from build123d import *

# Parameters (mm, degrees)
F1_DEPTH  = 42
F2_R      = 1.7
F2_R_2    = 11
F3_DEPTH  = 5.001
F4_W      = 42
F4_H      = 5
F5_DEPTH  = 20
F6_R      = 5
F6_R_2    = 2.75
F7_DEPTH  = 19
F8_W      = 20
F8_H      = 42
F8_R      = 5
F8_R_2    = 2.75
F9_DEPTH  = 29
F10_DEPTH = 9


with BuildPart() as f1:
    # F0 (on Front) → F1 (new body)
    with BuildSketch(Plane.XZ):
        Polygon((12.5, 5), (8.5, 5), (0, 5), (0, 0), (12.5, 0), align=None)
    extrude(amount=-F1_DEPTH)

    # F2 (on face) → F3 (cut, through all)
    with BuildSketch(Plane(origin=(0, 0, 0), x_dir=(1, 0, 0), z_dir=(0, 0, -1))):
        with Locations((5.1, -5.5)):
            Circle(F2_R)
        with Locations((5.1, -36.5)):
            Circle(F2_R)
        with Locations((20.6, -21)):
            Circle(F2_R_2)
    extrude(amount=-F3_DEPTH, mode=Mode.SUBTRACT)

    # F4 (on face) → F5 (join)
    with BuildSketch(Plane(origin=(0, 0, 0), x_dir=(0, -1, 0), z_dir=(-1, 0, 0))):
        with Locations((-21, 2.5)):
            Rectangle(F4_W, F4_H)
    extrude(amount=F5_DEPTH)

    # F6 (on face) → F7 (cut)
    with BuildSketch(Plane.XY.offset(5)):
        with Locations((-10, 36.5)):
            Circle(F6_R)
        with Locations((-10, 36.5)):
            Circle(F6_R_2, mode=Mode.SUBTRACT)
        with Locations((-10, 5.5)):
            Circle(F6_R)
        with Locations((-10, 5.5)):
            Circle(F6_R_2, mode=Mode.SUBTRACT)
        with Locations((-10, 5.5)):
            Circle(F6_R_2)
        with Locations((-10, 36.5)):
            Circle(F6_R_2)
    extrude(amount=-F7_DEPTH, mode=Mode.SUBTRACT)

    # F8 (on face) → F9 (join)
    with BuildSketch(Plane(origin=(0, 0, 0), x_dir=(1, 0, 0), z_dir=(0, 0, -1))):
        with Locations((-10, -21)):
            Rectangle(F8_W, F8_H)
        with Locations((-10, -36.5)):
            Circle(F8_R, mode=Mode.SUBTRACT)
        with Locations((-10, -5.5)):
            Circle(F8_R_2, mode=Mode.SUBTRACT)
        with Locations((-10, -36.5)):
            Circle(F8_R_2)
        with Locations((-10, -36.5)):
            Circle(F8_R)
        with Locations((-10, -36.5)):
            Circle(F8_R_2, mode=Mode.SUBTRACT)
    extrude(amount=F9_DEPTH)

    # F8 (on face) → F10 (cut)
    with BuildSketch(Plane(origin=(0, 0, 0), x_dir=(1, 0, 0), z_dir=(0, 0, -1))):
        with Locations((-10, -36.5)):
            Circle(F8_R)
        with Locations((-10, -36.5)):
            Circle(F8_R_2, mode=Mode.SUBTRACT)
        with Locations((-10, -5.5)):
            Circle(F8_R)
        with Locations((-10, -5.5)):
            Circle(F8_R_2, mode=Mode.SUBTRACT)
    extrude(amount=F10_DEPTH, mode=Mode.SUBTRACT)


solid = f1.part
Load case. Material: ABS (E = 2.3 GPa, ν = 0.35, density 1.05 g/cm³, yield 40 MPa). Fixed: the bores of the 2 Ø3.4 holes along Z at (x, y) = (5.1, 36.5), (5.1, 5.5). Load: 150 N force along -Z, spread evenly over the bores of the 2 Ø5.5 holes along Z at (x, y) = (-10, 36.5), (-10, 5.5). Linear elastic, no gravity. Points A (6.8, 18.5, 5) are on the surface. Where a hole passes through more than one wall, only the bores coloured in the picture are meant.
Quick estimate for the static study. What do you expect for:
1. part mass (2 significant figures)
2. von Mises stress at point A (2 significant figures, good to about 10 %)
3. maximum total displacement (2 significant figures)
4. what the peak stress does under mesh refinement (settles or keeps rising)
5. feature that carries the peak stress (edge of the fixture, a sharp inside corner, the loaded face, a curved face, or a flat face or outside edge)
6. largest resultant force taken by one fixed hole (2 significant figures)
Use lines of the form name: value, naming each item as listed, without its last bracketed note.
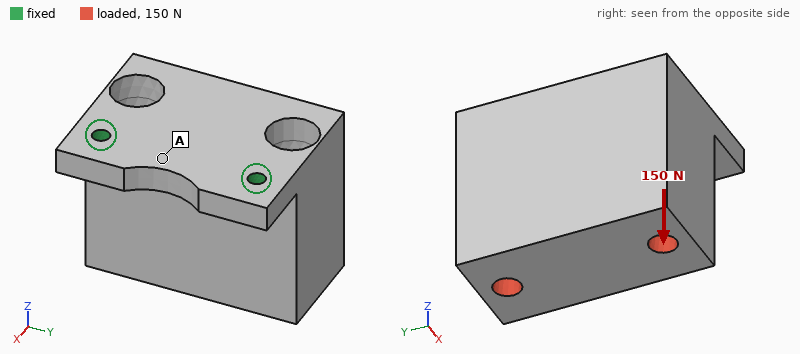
part mass: 29 g
von Mises stress at point A: 2.9 MPa
maximum total displacement: 0.67 mm
what the peak stress does under mesh refinement: keeps rising
feature that carries the peak stress: edge of the fixture
largest resultant force taken by one fixed hole: 75 N
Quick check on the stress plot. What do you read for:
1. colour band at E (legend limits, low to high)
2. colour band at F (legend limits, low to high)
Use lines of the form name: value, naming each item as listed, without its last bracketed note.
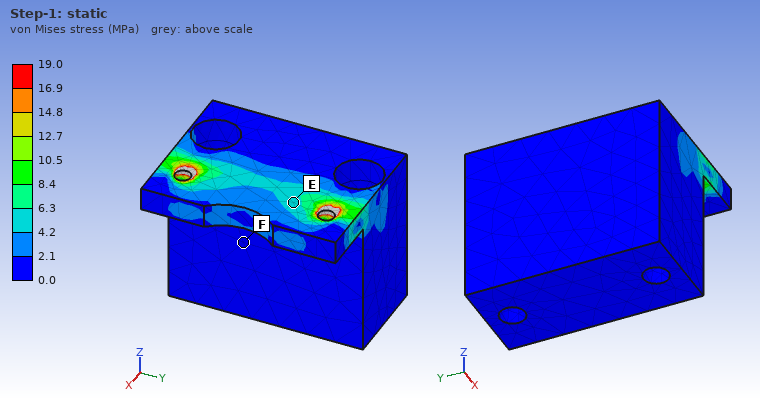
colour band at E: 4.2 to 6.3 MPa
colour band at F: 0.0 to 2.1 MPa
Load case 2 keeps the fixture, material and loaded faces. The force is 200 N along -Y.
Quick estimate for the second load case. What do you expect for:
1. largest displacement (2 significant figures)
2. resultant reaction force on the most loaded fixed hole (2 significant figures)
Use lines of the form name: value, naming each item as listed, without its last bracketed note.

largest displacement: 0.12 mm
resultant reaction force on the most loaded fixed hole: 190 N
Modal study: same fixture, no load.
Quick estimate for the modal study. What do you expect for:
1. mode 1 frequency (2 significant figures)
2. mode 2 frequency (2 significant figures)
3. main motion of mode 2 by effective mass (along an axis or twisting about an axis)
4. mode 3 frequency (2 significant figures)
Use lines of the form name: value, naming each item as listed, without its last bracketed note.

mode 1 frequency: 440 Hz
mode 2 frequency: 1700 Hz
main motion of mode 2 by effective mass: along Y
mode 3 frequency: 2900 Hz
